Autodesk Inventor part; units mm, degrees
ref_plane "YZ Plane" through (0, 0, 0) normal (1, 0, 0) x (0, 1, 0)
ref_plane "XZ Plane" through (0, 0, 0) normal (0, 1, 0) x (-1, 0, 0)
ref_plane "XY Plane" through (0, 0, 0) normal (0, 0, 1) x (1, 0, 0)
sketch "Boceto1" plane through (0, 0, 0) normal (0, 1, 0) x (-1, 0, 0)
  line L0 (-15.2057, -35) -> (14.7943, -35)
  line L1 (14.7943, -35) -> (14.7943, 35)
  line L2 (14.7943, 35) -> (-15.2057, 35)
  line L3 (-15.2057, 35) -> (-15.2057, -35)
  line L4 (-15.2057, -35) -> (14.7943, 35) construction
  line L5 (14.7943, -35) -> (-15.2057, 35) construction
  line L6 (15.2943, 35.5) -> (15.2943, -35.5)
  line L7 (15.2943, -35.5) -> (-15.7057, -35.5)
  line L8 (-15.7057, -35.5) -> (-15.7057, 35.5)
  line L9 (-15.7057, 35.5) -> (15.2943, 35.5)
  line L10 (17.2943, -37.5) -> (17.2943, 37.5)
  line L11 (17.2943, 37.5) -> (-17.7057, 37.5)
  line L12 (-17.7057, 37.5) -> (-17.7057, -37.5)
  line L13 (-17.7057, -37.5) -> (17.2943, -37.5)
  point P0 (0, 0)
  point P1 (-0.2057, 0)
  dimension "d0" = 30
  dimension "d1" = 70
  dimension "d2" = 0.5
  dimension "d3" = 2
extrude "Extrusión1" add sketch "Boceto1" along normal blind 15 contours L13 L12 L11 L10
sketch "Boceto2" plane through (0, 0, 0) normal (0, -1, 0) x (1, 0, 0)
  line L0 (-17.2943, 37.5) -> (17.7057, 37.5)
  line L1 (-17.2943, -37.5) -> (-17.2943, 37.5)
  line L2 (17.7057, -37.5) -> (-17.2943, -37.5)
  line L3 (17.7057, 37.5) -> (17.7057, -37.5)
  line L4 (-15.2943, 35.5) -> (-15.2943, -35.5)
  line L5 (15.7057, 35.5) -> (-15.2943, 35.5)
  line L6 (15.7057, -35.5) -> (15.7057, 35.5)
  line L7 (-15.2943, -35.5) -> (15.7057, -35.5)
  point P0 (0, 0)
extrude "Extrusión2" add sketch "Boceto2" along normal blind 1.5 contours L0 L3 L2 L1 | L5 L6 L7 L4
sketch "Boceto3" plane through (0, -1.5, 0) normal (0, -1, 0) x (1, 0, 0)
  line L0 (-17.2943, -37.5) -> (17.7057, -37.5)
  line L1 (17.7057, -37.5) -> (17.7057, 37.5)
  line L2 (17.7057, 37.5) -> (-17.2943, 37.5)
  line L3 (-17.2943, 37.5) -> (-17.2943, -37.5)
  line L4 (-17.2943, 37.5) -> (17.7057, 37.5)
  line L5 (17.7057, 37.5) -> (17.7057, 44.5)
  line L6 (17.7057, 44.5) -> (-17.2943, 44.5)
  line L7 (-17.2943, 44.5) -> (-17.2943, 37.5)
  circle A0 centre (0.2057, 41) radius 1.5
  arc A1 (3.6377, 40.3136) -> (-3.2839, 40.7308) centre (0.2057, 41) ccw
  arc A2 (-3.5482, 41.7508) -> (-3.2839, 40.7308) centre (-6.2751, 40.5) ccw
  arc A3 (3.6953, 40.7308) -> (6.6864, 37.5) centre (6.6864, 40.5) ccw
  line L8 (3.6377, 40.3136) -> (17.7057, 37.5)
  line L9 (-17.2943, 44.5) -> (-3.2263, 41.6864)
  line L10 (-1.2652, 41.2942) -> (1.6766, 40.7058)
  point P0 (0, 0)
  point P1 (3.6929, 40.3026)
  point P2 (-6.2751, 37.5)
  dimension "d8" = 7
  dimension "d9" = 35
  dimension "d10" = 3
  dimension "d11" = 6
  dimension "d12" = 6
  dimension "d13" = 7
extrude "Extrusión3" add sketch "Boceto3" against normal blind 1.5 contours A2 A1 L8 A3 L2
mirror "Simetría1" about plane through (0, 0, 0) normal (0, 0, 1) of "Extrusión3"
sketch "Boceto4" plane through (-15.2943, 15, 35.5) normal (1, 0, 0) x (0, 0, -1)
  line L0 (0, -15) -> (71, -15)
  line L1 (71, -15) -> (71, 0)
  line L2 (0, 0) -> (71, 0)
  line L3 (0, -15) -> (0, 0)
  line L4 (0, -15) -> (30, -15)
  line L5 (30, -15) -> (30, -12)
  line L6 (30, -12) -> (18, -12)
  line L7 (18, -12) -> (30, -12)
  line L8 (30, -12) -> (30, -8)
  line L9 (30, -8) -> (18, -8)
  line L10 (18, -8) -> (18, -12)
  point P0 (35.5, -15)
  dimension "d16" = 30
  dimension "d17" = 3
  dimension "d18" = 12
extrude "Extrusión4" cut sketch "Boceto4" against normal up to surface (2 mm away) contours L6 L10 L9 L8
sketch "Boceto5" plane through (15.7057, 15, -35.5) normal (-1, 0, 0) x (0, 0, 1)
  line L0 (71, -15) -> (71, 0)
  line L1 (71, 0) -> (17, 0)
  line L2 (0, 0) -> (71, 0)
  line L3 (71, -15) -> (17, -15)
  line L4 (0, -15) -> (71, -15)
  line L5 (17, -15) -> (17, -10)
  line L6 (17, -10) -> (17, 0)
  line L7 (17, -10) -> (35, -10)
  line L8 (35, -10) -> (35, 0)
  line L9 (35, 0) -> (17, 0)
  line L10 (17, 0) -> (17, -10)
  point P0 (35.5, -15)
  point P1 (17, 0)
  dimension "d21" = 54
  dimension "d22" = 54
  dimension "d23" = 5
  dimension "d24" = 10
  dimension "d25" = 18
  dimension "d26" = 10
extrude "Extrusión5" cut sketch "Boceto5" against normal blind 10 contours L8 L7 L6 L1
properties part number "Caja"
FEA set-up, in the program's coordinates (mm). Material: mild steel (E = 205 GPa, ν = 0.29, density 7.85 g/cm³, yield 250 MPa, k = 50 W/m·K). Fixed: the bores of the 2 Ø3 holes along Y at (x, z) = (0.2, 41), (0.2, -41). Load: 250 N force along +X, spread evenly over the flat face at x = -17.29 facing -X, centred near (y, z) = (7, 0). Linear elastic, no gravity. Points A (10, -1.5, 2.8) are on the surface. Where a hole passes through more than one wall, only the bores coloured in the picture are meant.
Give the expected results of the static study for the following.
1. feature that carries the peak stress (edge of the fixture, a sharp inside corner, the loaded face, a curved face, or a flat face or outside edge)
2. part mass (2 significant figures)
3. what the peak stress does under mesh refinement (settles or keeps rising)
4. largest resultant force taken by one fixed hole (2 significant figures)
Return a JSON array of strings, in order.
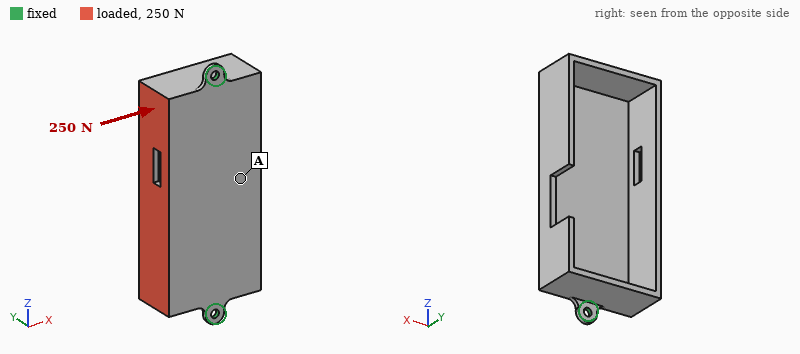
["edge of the fixture", "78 g", "keeps rising", "130 N"]
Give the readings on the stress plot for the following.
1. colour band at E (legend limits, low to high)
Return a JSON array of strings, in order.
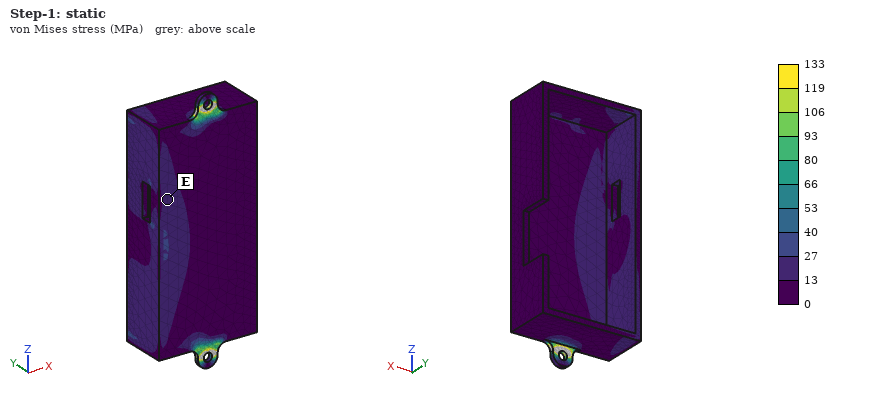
["13 to 27 MPa"]
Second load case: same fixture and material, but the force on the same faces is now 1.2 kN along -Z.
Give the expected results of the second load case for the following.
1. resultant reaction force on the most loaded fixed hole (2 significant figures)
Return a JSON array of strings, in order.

["660 N"]
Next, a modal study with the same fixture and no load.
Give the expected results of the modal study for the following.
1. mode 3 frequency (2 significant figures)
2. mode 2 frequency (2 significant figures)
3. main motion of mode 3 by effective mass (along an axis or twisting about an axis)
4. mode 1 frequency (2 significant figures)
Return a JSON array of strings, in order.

["2800 Hz", "2100 Hz", "along Y", "1000 Hz"]
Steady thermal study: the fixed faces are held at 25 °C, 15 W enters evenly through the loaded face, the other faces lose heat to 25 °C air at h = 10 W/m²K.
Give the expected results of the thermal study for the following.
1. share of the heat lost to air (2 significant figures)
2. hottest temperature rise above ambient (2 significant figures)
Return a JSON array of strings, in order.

["35 %", "89 K"]
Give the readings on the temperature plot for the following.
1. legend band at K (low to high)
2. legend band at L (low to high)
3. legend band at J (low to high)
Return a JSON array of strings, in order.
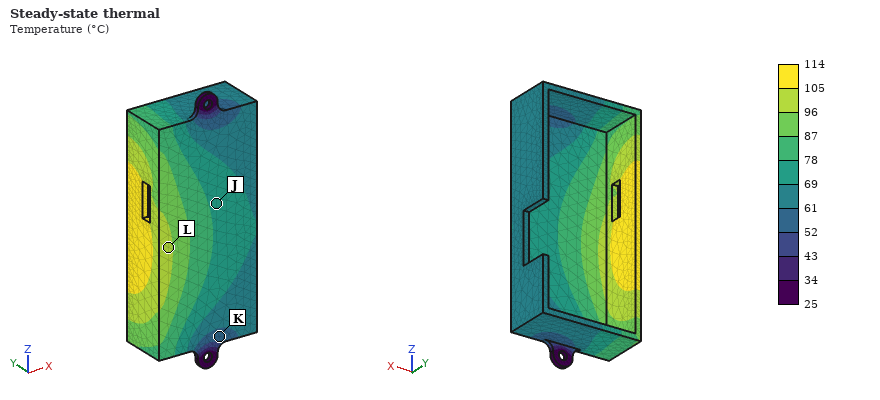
["52 to 61 °C", "96 to 105 °C", "69 to 78 °C"]
